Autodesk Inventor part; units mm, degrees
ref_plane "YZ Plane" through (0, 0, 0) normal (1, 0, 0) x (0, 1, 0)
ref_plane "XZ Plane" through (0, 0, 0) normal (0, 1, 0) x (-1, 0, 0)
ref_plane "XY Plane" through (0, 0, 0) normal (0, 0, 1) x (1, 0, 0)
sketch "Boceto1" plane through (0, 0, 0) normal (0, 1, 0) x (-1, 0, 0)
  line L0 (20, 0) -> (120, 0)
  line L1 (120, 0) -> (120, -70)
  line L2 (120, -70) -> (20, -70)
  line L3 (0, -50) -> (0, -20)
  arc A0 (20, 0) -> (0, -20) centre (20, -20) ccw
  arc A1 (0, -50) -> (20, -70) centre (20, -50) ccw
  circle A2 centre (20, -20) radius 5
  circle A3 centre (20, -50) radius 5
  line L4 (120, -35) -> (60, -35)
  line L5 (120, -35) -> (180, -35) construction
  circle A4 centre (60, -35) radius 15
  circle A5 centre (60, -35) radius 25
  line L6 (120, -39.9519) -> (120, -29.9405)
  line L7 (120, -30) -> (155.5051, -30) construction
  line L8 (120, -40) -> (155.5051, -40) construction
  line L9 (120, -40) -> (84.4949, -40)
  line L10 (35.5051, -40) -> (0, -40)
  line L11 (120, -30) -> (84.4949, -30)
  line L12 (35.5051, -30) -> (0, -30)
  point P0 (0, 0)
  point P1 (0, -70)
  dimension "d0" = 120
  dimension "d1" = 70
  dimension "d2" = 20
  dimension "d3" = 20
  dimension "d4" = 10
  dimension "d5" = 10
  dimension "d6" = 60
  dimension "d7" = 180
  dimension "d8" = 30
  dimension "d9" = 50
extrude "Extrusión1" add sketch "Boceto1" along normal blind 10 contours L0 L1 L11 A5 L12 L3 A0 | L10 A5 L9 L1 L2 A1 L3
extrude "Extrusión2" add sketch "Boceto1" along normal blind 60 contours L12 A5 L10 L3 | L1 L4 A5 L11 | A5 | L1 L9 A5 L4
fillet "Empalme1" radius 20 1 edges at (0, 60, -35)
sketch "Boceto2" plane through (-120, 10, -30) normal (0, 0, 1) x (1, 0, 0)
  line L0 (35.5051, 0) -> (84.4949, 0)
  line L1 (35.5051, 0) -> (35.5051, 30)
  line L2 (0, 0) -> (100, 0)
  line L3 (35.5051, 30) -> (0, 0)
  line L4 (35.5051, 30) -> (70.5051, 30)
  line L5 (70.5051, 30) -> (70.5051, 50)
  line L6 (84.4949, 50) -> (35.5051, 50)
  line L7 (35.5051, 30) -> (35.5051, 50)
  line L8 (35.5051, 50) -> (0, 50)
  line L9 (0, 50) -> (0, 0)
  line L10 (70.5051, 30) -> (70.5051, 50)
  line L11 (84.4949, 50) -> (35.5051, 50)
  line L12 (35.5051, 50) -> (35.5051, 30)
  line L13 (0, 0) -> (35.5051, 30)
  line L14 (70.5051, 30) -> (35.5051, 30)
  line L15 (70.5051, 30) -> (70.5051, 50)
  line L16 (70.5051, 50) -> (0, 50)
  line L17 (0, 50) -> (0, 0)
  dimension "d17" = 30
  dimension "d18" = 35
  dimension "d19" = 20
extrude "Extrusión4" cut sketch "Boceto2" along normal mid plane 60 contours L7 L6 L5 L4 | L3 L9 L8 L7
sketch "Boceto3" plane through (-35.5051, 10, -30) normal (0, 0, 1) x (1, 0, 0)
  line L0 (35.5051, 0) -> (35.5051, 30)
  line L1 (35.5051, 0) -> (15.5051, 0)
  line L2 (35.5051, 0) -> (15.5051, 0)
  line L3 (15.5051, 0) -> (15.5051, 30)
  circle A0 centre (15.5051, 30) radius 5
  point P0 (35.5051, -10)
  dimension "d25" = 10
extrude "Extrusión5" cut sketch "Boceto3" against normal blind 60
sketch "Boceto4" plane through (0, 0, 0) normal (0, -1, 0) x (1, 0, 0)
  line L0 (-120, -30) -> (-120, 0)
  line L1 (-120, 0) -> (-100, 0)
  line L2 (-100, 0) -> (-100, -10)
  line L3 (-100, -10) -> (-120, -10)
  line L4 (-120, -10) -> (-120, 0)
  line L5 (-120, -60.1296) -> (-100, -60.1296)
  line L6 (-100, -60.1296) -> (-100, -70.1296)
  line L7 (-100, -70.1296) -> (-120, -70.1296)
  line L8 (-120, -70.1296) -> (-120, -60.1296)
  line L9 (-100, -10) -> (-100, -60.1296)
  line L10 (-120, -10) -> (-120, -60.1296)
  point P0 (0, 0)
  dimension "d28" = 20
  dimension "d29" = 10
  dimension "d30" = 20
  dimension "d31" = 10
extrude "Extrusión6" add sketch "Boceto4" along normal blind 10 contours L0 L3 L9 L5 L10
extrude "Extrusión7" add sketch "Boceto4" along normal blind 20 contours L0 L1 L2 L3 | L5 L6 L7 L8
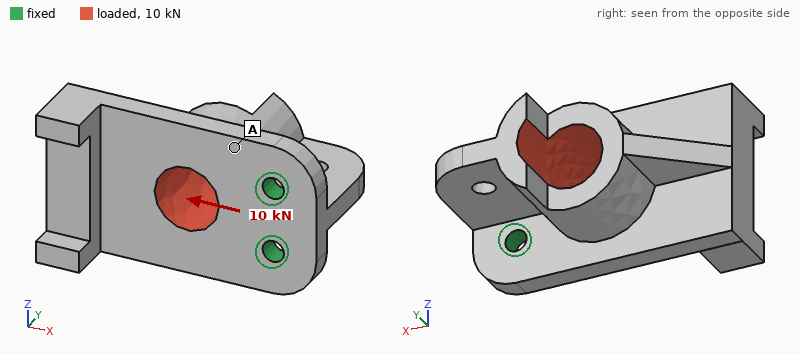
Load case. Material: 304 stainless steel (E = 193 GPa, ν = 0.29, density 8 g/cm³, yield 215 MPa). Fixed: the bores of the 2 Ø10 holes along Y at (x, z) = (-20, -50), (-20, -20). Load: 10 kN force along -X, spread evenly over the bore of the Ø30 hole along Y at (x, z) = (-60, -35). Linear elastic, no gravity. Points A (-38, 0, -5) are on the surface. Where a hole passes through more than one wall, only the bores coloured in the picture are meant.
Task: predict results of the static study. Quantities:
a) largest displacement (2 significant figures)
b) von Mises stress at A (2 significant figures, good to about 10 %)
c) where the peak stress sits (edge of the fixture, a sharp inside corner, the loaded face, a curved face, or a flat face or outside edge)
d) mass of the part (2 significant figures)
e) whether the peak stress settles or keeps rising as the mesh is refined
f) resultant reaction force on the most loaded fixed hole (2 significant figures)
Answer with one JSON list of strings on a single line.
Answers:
["0.11 mm", "21 MPa", "edge of the fixture", "1.3 kg", "keeps rising", "5.0 kN"]
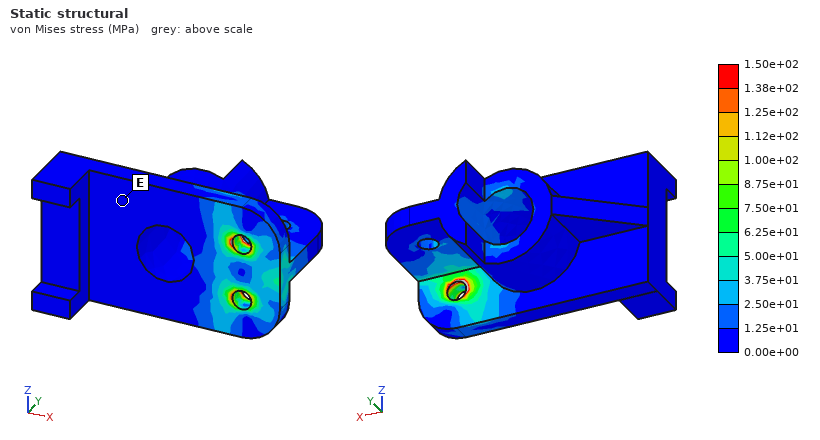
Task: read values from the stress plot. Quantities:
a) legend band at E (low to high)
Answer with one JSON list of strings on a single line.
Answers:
["0.00e+00 to 1.25e+01 MPa"]
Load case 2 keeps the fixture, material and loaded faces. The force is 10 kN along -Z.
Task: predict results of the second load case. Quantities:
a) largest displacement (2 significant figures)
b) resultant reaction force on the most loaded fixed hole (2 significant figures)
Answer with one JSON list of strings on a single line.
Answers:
["59 µm", "12 kN"]
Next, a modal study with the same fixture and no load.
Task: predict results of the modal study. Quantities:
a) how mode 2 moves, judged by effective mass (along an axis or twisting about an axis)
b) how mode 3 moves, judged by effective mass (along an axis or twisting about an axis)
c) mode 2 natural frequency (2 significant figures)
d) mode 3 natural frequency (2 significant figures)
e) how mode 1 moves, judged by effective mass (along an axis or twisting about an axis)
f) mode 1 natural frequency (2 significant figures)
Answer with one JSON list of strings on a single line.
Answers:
["along Z", "along Z", "2200 Hz", "2500 Hz", "along Y", "1000 Hz"]
